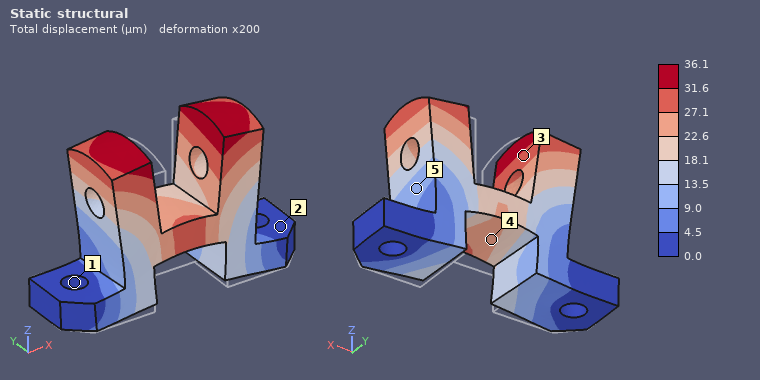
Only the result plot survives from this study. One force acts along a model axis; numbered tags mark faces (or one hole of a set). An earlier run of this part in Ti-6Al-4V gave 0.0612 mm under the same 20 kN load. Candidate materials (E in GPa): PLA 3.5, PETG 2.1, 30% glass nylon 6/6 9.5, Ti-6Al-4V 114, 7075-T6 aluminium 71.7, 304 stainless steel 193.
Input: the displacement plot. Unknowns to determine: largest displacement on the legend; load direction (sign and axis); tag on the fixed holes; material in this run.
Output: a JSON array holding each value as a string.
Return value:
["36.1 µm", "+Z", "1", "304 stainless steel"]
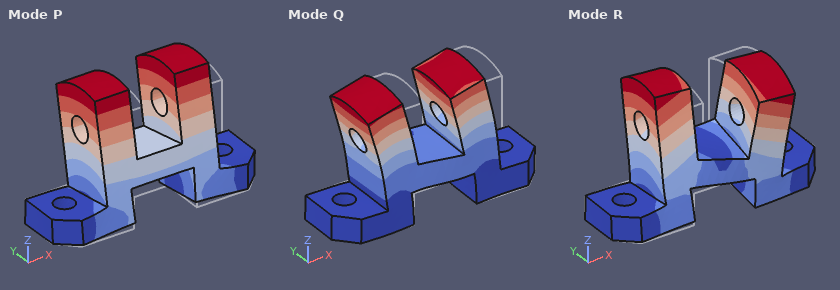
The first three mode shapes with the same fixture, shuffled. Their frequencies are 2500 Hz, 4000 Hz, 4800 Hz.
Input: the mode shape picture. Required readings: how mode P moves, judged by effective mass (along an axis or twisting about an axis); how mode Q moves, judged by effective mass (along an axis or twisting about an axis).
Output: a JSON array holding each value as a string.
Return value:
["along Y", "along X"]
